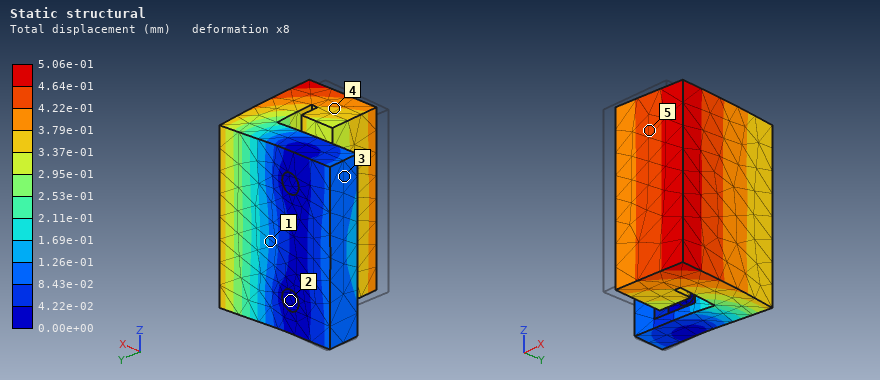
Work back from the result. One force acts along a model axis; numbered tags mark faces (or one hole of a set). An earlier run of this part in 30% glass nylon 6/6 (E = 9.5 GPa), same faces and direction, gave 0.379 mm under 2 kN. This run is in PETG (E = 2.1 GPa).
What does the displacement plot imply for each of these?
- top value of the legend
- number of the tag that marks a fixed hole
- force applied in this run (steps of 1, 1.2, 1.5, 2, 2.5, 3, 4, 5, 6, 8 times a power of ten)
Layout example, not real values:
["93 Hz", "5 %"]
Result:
["5.06e-01 mm", "2", "600 N"]
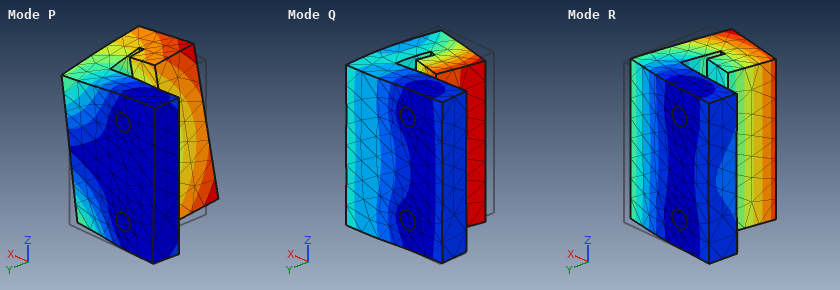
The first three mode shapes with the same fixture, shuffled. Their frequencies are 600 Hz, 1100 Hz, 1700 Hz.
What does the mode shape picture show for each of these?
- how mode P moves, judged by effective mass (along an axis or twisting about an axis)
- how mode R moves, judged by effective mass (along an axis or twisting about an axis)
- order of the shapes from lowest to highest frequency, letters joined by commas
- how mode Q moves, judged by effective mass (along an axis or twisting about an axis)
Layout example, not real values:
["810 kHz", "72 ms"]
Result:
["along Z", "along X", "R, P, Q", "along Y"]
